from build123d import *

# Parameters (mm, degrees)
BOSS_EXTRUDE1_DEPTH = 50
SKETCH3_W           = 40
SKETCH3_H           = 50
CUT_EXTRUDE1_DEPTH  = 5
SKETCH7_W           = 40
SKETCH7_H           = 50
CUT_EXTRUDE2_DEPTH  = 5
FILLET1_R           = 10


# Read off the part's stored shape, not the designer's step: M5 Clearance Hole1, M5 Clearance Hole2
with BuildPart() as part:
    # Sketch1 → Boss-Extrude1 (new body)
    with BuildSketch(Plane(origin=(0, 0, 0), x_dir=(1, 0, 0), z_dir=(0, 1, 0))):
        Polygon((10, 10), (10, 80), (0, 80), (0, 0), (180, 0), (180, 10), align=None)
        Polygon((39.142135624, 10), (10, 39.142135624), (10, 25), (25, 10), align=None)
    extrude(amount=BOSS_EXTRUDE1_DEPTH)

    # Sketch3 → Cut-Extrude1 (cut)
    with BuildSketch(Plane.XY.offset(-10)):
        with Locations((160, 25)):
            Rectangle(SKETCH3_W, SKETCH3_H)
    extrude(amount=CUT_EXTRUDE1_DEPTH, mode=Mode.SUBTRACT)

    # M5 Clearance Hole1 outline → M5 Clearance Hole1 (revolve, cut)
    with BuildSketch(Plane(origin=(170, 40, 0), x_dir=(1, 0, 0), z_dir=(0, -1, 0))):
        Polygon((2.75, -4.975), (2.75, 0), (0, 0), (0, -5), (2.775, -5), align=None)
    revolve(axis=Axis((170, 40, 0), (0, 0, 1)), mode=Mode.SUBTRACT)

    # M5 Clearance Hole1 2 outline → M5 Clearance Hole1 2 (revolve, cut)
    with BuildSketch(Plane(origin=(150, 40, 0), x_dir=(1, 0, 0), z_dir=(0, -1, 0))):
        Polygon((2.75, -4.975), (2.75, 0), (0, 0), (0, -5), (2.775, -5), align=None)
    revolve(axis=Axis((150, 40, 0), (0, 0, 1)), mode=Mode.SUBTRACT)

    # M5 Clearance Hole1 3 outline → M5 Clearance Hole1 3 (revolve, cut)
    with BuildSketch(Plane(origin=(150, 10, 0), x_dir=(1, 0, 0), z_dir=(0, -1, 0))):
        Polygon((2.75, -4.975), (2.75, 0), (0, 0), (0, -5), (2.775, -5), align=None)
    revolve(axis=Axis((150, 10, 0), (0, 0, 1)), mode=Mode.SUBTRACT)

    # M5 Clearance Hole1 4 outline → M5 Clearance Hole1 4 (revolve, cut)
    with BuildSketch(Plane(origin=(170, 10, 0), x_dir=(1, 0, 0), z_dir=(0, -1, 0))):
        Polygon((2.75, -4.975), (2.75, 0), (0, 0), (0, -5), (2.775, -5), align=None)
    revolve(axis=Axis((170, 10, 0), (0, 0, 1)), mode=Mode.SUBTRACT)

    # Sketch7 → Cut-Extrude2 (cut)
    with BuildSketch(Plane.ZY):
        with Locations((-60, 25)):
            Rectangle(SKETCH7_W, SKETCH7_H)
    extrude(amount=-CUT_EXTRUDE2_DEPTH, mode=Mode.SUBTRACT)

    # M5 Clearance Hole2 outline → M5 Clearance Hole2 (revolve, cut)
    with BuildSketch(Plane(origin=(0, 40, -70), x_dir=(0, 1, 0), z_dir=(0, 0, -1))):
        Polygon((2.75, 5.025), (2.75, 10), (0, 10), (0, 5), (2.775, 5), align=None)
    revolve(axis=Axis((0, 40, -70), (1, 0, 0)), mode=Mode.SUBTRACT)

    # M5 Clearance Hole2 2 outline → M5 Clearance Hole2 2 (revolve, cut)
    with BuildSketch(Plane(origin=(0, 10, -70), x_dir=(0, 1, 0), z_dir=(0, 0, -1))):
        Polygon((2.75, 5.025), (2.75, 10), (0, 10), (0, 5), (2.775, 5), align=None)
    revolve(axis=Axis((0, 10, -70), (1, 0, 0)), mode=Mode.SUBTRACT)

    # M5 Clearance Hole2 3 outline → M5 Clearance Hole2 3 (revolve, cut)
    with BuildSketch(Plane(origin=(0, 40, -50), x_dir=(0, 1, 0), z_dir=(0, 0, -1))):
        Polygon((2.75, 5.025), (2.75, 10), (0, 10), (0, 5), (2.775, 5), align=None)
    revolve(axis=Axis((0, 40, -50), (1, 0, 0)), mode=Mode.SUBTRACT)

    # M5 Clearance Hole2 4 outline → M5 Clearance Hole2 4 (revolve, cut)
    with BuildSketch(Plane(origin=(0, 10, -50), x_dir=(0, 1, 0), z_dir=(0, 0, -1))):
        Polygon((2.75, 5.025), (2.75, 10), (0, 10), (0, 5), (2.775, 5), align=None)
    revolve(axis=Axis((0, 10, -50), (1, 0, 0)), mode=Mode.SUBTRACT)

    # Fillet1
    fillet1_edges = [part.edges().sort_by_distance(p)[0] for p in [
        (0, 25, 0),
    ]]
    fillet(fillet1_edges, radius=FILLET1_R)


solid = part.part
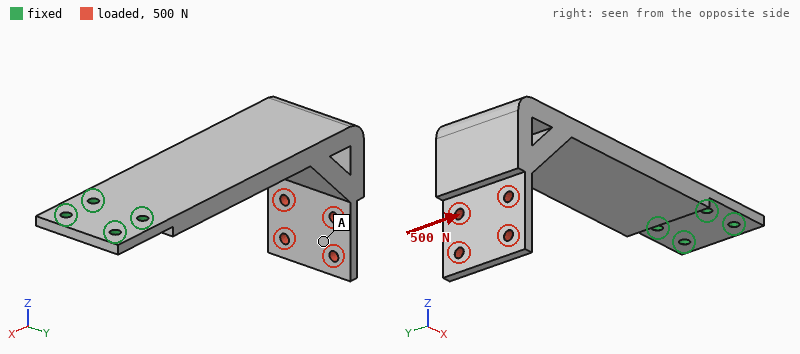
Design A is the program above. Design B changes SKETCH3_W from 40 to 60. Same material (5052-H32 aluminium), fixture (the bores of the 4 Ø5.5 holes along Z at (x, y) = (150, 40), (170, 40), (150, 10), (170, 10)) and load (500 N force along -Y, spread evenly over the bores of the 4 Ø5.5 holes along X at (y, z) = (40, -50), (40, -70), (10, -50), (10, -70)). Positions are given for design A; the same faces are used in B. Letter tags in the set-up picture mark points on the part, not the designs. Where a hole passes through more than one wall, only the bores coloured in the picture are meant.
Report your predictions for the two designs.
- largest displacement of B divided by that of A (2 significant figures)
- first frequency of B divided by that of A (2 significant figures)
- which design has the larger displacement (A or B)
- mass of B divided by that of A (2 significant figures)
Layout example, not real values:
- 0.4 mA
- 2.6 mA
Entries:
- 1.2
- 0.84
- B
- 0.98
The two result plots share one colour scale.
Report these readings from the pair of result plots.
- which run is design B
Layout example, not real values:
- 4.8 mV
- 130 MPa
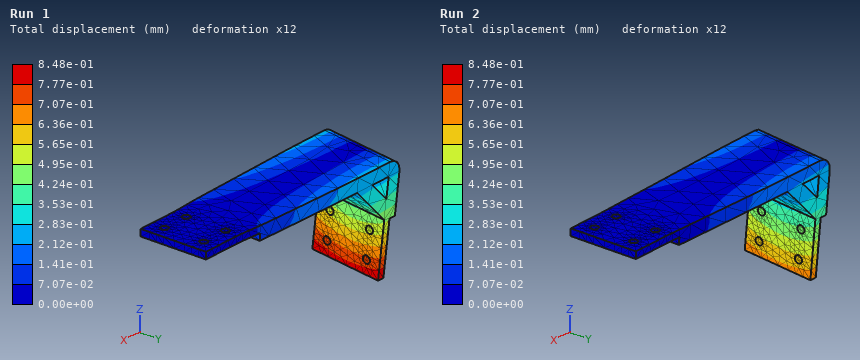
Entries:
- Run 1
